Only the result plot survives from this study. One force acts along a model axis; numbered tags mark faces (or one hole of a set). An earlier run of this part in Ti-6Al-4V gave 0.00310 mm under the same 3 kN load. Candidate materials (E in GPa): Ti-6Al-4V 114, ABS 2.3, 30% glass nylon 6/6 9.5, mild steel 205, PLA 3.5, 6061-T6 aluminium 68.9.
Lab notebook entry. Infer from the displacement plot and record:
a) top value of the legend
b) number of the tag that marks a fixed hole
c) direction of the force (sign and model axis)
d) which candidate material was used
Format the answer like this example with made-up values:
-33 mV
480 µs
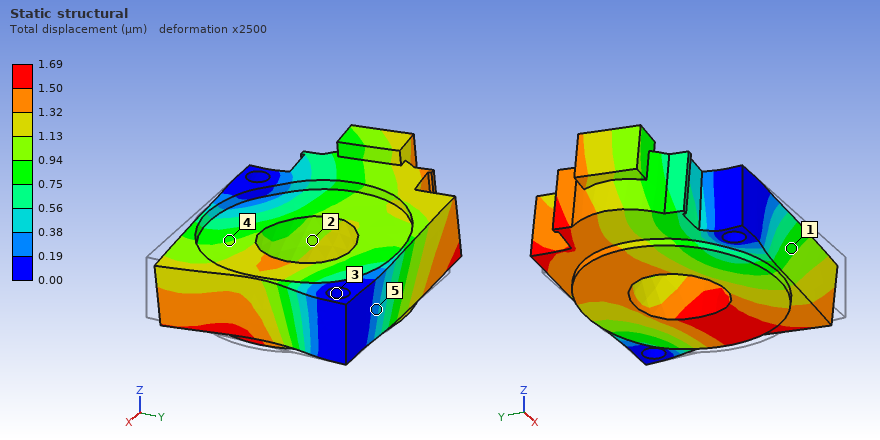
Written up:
1.69 µm
3
-X
mild steel
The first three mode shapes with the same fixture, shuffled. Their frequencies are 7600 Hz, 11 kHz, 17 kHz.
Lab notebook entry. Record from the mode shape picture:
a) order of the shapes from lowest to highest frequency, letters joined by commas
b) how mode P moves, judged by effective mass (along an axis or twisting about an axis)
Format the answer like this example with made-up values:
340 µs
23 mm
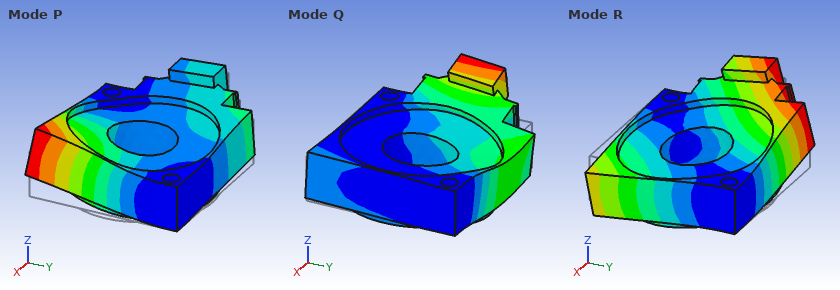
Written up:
R, P, Q
along Z
